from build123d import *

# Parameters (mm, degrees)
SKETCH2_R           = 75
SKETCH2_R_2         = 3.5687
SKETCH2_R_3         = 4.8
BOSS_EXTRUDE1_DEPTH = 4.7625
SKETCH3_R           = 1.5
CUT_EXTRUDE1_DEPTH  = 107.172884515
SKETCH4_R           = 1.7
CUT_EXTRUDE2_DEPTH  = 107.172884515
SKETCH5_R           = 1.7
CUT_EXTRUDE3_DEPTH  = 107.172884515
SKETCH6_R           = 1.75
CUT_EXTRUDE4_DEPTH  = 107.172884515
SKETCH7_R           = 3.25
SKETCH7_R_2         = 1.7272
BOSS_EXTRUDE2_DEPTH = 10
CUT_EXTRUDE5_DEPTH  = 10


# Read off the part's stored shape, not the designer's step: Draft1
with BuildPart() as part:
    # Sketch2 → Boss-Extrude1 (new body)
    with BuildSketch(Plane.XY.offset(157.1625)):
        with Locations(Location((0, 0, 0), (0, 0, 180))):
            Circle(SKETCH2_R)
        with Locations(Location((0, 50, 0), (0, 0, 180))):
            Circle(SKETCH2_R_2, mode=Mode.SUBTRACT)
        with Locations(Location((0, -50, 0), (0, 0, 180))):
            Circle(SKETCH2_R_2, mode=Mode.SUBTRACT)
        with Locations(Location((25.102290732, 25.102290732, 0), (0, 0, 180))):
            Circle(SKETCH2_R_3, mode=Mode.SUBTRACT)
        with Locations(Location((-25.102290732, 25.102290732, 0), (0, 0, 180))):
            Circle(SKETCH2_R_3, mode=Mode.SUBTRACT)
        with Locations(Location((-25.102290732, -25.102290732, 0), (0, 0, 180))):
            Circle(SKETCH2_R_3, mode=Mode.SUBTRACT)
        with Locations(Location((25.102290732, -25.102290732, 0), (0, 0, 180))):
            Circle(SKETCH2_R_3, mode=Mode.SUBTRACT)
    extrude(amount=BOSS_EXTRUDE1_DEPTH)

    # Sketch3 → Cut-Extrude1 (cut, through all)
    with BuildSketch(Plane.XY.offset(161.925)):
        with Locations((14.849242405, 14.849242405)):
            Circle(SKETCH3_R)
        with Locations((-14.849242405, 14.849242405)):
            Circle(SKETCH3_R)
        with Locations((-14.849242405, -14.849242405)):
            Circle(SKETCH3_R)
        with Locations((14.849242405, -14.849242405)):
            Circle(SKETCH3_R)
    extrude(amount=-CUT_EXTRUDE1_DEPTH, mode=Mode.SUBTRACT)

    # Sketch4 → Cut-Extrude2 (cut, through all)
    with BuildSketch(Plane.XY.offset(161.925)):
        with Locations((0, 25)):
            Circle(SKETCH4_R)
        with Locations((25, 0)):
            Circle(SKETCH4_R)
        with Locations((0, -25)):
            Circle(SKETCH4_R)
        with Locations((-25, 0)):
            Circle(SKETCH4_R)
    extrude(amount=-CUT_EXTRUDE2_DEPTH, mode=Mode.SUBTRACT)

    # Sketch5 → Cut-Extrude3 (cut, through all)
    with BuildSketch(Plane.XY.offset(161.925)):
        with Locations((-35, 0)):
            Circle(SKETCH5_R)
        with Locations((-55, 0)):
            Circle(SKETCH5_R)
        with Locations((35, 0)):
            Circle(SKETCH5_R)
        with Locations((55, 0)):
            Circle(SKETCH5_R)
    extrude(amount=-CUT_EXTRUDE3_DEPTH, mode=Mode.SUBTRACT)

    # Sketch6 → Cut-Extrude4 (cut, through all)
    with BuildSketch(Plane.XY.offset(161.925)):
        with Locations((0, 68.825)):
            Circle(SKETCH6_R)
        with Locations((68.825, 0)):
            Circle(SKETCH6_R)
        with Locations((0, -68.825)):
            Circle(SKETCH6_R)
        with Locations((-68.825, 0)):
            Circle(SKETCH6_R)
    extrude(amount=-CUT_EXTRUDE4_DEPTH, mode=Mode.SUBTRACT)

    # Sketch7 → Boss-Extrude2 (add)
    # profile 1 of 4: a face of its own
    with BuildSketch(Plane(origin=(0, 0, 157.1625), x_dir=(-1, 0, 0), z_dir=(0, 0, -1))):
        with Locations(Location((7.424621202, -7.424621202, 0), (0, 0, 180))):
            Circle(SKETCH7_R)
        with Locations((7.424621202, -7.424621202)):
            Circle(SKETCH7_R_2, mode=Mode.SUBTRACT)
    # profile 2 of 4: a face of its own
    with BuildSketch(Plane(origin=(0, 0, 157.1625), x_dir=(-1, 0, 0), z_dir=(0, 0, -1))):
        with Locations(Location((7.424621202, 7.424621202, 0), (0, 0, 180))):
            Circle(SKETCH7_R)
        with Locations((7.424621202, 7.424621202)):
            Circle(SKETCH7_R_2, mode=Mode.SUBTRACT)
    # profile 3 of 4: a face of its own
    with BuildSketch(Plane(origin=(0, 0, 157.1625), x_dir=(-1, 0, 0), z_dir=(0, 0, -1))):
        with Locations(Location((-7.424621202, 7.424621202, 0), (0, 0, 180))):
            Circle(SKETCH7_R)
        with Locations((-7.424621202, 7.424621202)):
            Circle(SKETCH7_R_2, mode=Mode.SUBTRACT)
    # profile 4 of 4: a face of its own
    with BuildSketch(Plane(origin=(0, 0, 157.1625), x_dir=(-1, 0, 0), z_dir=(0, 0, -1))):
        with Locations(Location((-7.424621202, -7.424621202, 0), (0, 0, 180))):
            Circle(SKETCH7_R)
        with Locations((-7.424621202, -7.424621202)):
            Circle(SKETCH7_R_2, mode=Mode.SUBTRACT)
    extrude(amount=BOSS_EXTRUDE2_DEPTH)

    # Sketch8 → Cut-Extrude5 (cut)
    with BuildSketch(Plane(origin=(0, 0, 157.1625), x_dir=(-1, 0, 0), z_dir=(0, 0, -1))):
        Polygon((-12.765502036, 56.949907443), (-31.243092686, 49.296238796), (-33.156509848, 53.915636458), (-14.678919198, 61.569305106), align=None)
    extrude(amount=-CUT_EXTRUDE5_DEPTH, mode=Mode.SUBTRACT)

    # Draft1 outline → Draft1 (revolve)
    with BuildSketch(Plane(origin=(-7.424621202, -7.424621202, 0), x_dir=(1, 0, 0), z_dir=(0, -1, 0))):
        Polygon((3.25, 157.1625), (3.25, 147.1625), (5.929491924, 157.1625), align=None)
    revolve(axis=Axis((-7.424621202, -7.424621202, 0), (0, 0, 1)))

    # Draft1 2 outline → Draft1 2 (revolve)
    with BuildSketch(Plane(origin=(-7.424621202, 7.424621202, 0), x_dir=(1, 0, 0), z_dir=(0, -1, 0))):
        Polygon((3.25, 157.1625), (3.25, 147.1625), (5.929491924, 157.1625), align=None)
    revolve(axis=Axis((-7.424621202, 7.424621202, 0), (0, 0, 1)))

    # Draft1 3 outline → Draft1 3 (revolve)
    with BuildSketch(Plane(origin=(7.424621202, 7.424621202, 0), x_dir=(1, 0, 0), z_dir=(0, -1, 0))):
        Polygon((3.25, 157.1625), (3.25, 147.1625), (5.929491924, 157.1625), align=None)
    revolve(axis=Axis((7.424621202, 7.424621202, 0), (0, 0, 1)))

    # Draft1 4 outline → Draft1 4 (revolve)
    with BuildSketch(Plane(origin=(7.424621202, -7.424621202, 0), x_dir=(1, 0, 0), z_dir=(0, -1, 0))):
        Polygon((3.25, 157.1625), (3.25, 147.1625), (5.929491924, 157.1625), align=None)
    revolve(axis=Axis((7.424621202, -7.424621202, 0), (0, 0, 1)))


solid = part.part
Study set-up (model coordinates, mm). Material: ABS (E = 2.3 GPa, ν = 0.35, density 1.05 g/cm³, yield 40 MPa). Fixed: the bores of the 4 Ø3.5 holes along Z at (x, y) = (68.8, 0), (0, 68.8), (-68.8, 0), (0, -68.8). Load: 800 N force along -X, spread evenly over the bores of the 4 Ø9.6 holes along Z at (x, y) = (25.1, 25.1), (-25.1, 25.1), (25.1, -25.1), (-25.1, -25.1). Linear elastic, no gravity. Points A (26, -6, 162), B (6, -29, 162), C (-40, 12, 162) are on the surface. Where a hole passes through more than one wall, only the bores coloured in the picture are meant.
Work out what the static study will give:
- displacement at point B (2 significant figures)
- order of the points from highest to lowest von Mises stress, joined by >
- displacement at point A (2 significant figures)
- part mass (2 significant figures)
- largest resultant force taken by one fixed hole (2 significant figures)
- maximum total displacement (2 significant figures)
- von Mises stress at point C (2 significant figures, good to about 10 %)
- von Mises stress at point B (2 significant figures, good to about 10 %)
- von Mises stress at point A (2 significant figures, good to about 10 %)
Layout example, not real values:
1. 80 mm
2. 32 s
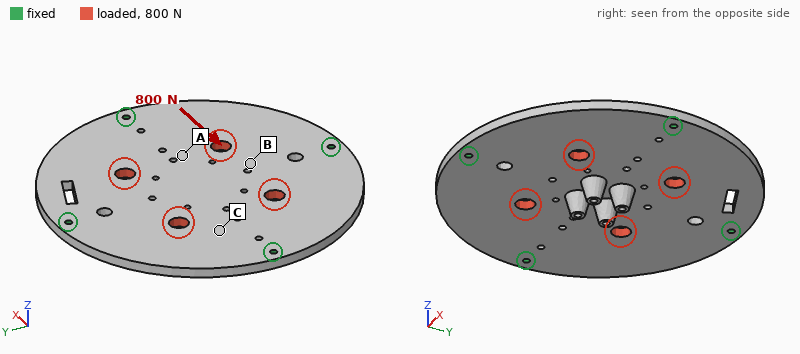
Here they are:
1. 37 µm
2. C > A > B
3. 34 µm
4. 88 g
5. 230 N
6. 44 µm
7. 1.3 MPa
8. 0.34 MPa
9. 0.68 MPa
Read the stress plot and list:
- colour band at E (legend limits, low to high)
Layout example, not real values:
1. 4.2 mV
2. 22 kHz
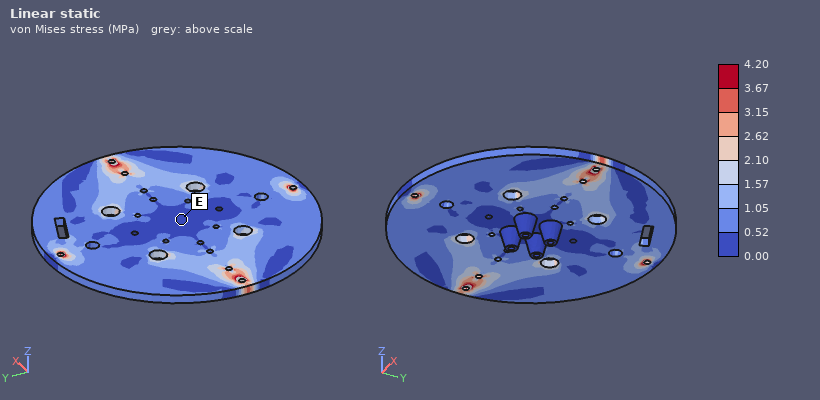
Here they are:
1. 0.00 to 0.52 MPa
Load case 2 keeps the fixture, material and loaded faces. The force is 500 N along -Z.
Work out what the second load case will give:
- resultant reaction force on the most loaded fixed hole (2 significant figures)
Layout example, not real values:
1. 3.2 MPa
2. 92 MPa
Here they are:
1. 130 N
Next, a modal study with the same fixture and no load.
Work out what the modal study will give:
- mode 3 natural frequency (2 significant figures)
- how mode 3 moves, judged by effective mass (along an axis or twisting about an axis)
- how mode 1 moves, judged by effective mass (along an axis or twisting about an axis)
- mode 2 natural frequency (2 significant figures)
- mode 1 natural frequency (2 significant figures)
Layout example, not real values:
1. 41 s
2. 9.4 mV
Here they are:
1. 630 Hz
2. twisting about X
3. along Z
4. 590 Hz
5. 460 Hz
